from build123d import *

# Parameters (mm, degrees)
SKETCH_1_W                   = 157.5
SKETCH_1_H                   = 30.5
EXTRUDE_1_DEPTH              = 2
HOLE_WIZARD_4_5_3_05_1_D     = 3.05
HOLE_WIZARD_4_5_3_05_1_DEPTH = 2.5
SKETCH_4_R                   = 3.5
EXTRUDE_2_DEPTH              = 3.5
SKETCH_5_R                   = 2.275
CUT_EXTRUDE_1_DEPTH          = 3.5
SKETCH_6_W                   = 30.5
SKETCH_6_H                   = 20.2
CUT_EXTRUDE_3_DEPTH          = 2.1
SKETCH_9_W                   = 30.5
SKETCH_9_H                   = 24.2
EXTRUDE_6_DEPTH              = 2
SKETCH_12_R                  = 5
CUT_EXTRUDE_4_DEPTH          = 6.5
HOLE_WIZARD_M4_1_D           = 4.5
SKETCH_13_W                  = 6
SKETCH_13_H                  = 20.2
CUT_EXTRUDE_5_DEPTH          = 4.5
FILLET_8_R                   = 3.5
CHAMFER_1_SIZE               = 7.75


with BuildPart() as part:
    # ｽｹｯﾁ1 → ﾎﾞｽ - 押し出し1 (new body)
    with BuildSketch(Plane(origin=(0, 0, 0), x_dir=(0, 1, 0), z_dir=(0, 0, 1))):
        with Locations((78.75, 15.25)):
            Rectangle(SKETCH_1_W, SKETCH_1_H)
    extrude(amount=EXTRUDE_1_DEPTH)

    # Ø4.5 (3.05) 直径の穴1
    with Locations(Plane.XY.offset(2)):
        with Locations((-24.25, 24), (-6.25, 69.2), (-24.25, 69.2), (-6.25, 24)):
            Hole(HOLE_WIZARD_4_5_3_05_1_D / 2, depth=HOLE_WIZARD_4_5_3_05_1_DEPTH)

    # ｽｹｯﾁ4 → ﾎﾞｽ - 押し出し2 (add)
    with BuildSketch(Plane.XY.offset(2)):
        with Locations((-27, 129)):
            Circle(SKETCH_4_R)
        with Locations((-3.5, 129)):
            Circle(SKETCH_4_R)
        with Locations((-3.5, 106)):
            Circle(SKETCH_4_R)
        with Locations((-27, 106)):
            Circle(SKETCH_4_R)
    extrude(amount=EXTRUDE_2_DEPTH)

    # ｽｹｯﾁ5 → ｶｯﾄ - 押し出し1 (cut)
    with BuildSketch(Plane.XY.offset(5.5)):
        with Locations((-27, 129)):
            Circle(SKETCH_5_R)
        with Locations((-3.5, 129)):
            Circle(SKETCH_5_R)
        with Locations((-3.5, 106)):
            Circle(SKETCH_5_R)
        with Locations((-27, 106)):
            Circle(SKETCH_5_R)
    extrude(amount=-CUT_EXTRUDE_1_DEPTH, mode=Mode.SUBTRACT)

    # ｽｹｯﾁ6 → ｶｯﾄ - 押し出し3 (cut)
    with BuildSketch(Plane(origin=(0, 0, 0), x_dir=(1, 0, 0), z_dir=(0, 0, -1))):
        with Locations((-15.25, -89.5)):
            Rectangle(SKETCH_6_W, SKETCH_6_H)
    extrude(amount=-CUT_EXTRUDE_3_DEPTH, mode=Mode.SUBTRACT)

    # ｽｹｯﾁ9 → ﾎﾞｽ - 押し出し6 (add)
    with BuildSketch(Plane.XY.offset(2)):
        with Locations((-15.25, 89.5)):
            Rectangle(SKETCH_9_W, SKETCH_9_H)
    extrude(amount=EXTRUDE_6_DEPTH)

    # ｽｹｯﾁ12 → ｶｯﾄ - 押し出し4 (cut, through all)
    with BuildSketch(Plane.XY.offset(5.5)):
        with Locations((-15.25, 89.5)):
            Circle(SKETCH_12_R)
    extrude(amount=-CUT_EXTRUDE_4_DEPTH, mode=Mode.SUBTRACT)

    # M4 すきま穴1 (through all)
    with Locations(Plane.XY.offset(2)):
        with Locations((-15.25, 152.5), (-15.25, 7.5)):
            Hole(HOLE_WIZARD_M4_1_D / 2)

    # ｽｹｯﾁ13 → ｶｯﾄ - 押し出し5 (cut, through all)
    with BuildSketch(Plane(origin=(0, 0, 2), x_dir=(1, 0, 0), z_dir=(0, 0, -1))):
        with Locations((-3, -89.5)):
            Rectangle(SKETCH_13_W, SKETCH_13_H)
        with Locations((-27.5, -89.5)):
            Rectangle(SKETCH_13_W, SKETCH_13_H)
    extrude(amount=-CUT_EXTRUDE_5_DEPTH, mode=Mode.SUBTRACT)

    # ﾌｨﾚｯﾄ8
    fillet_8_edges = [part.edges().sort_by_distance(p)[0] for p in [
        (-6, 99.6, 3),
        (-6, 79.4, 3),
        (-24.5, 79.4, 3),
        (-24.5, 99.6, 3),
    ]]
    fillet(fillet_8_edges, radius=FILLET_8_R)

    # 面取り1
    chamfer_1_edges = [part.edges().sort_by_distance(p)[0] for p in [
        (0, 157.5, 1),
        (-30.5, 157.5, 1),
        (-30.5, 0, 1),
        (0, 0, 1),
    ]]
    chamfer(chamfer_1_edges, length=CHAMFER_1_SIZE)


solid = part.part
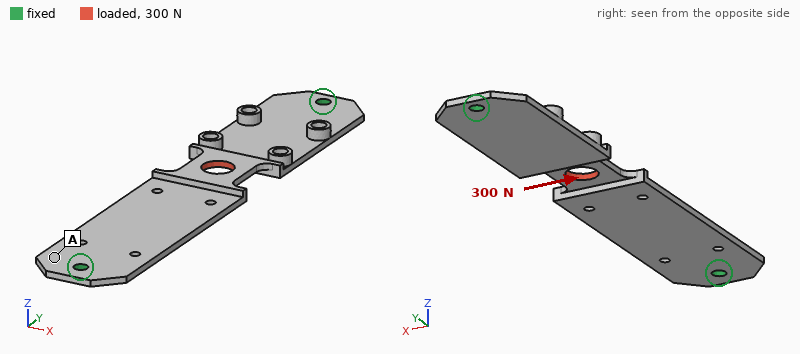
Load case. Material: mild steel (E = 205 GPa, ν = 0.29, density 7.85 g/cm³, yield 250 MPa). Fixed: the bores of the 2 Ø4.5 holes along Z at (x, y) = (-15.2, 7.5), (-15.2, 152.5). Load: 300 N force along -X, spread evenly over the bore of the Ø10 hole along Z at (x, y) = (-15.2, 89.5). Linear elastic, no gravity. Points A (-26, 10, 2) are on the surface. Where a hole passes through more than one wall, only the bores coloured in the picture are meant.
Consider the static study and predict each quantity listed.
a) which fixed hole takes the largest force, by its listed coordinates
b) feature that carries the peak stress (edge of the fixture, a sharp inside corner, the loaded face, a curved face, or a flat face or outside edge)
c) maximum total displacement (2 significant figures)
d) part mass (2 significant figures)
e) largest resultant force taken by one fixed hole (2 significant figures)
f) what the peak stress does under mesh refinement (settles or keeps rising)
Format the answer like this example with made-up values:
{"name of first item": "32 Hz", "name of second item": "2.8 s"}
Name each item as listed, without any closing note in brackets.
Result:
{"which fixed hole takes the largest force, by its listed coordinates": "(-15.2, 152.5)", "feature that carries the peak stress": "edge of the fixture", "maximum total displacement": "70 µm", "part mass": "72 g", "largest resultant force taken by one fixed hole": "180 N", "what the peak stress does under mesh refinement": "keeps rising"}
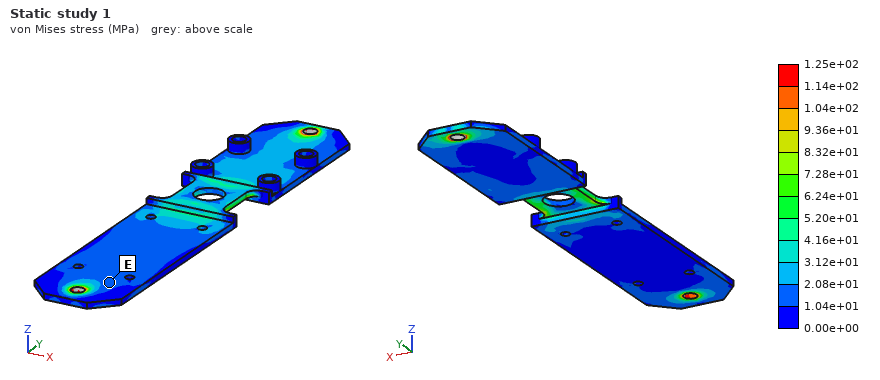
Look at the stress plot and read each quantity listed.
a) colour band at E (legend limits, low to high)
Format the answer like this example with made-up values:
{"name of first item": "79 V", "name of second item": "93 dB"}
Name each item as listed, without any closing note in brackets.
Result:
{"colour band at E": "1.04e+01 to 2.08e+01 MPa"}
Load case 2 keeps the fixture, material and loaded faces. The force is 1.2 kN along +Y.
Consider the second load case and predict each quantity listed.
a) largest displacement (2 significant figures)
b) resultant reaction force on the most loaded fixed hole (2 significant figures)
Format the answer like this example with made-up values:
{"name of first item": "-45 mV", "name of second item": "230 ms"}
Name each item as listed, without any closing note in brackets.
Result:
{"largest displacement": "98 µm", "resultant reaction force on the most loaded fixed hole": "600 N"}
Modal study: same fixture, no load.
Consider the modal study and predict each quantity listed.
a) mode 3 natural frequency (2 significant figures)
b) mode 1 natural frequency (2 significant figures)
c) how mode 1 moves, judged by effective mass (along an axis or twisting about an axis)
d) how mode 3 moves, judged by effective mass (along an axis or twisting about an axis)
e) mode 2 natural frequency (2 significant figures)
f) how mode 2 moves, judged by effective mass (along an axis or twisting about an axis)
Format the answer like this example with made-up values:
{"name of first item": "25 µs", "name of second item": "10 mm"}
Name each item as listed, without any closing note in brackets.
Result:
{"mode 3 natural frequency": "1500 Hz", "mode 1 natural frequency": "530 Hz", "how mode 1 moves, judged by effective mass": "along Z", "how mode 3 moves, judged by effective mass": "twisting about Y", "mode 2 natural frequency": "1300 Hz", "how mode 2 moves, judged by effective mass": "twisting about X"}
